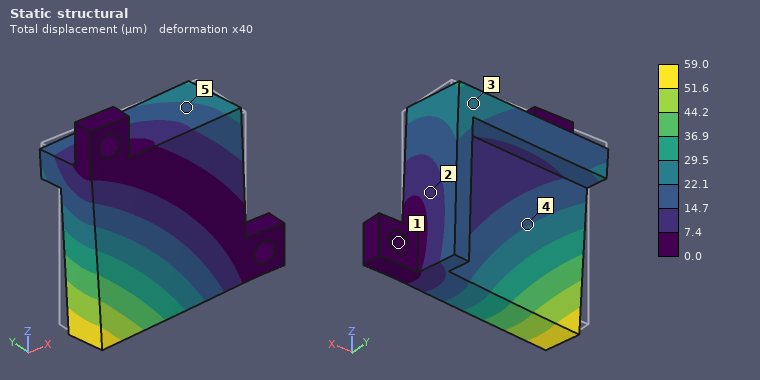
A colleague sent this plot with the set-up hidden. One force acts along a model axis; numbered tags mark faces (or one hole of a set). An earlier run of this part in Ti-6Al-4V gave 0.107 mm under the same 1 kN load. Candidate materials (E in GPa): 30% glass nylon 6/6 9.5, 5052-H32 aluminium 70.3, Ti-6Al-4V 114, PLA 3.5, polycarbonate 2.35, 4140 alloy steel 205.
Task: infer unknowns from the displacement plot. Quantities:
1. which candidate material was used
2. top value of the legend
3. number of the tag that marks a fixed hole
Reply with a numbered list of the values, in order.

1. 4140 alloy steel
2. 59.0 µm
3. 1
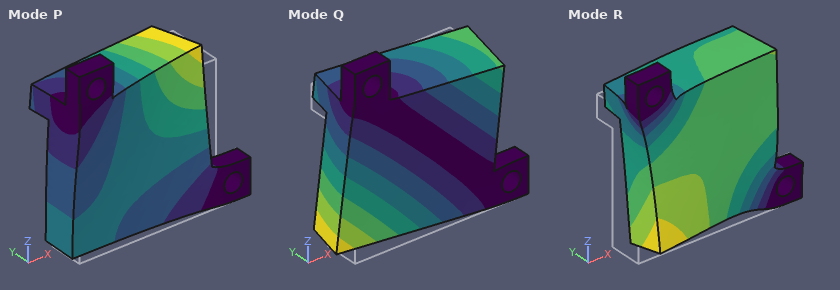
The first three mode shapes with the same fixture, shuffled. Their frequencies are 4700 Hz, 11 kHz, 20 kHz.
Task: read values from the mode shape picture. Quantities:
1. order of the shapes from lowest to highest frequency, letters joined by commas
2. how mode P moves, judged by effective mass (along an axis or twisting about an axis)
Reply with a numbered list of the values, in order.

1. Q, P, R
2. along Y
